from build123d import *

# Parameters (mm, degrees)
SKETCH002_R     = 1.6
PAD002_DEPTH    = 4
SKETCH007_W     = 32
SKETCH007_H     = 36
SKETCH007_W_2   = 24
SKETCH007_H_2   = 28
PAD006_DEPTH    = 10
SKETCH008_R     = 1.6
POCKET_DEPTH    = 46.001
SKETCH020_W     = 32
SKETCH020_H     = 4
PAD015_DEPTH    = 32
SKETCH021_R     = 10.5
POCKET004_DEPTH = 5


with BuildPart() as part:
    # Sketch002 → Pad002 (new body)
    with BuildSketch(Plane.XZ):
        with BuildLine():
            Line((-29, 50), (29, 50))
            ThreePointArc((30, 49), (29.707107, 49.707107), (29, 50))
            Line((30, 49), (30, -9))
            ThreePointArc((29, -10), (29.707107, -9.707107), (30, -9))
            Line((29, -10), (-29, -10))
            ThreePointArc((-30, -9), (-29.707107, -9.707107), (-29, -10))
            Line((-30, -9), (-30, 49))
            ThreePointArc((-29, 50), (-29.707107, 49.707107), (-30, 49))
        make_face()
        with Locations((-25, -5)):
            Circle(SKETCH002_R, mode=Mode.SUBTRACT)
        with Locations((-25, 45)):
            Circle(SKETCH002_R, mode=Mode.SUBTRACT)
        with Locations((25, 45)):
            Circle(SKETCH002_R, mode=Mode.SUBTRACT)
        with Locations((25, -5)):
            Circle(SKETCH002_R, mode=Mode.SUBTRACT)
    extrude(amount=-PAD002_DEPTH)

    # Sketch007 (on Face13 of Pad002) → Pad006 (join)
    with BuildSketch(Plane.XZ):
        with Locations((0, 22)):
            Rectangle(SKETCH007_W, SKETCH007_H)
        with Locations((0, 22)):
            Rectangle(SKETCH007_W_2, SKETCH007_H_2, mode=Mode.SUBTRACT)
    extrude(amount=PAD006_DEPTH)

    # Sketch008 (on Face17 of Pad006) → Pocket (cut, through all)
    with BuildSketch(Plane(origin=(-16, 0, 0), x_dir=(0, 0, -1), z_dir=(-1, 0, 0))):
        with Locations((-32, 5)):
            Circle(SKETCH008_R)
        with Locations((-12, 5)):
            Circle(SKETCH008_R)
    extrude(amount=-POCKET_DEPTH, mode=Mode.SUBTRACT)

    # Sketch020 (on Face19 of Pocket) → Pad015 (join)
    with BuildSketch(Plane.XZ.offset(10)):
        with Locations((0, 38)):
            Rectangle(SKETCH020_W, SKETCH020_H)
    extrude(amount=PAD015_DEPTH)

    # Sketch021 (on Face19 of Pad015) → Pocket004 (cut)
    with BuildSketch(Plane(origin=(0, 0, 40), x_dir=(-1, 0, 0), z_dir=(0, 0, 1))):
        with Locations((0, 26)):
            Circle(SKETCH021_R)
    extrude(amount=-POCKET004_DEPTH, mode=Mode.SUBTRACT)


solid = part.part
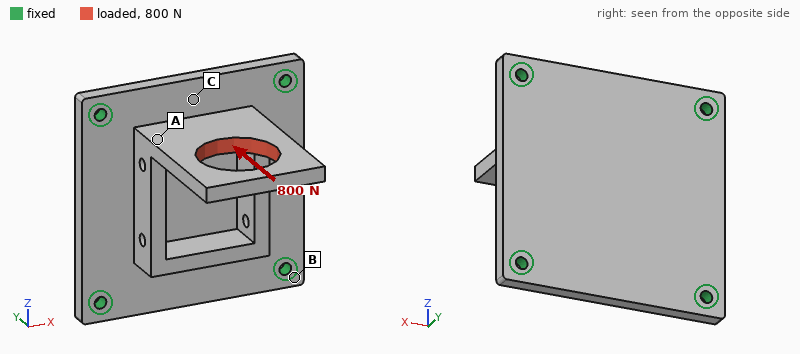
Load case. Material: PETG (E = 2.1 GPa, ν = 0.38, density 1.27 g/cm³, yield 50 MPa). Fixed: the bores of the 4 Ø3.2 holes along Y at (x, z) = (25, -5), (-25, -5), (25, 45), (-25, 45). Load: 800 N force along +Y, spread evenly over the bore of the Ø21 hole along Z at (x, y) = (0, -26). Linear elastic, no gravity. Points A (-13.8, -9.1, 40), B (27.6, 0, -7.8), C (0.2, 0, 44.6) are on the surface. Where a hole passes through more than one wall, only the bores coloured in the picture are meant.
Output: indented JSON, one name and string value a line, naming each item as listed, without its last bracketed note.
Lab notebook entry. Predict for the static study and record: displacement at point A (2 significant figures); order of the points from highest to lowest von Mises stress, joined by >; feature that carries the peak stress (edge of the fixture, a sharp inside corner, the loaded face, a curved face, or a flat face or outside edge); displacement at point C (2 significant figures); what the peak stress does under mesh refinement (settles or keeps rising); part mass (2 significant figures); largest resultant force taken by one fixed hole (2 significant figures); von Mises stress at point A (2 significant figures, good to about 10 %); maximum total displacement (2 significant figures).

{
  "displacement at point A": "0.64 mm",
  "order of the points from highest to lowest von Mises stress, joined by >": "A > C > B",
  "feature that carries the peak stress": "edge of the fixture",
  "displacement at point C": "0.65 mm",
  "what the peak stress does under mesh refinement": "keeps rising",
  "part mass": "27 g",
  "largest resultant force taken by one fixed hole": "370 N",
  "von Mises stress at point A": "14 MPa",
  "maximum total displacement": "1.1 mm"
}
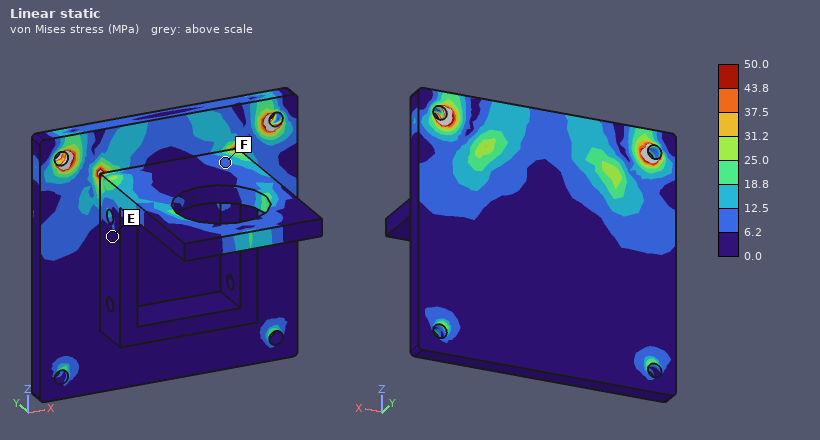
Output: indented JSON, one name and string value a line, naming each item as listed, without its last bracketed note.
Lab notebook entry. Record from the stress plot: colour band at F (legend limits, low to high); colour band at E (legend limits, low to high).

{
  "colour band at F": "6.2 to 12.5 MPa",
  "colour band at E": "0.0 to 6.2 MPa"
}
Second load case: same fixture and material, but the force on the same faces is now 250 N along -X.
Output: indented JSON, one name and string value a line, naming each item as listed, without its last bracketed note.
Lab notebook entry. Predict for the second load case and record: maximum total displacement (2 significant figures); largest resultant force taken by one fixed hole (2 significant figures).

{
  "maximum total displacement": "1.0 mm",
  "largest resultant force taken by one fixed hole": "180 N"
}
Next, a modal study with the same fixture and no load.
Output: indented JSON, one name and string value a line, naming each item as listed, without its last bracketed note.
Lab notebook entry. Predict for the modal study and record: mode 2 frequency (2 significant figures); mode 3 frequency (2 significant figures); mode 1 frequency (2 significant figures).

{
  "mode 2 frequency": "1300 Hz",
  "mode 3 frequency": "1500 Hz",
  "mode 1 frequency": "560 Hz"
}
